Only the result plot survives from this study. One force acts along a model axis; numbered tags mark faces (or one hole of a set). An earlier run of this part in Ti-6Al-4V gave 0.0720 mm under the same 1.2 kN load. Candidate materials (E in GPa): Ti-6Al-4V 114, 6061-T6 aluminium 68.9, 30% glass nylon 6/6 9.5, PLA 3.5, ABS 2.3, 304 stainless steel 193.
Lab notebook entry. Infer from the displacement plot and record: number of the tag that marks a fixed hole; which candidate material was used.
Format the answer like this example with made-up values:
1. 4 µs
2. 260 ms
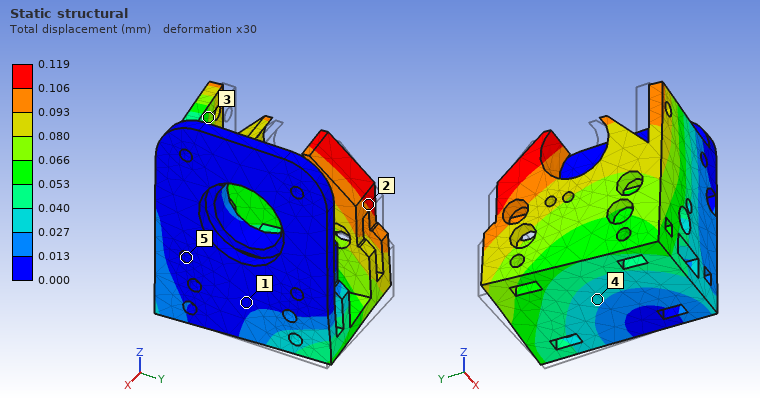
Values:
1. 5
2. 6061-T6 aluminium
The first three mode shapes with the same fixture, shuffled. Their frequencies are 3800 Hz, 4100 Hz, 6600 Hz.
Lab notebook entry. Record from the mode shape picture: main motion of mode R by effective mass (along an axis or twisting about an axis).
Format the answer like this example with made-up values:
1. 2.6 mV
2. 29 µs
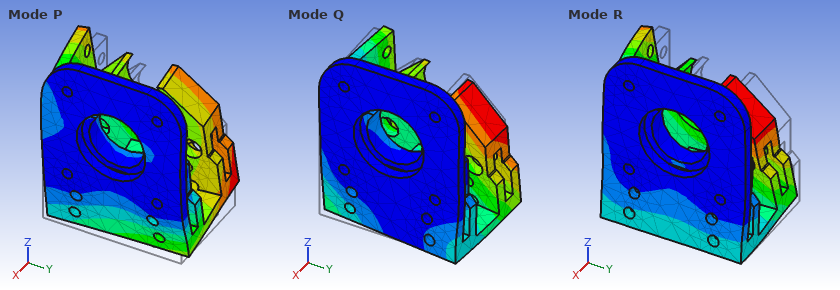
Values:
1. along X
